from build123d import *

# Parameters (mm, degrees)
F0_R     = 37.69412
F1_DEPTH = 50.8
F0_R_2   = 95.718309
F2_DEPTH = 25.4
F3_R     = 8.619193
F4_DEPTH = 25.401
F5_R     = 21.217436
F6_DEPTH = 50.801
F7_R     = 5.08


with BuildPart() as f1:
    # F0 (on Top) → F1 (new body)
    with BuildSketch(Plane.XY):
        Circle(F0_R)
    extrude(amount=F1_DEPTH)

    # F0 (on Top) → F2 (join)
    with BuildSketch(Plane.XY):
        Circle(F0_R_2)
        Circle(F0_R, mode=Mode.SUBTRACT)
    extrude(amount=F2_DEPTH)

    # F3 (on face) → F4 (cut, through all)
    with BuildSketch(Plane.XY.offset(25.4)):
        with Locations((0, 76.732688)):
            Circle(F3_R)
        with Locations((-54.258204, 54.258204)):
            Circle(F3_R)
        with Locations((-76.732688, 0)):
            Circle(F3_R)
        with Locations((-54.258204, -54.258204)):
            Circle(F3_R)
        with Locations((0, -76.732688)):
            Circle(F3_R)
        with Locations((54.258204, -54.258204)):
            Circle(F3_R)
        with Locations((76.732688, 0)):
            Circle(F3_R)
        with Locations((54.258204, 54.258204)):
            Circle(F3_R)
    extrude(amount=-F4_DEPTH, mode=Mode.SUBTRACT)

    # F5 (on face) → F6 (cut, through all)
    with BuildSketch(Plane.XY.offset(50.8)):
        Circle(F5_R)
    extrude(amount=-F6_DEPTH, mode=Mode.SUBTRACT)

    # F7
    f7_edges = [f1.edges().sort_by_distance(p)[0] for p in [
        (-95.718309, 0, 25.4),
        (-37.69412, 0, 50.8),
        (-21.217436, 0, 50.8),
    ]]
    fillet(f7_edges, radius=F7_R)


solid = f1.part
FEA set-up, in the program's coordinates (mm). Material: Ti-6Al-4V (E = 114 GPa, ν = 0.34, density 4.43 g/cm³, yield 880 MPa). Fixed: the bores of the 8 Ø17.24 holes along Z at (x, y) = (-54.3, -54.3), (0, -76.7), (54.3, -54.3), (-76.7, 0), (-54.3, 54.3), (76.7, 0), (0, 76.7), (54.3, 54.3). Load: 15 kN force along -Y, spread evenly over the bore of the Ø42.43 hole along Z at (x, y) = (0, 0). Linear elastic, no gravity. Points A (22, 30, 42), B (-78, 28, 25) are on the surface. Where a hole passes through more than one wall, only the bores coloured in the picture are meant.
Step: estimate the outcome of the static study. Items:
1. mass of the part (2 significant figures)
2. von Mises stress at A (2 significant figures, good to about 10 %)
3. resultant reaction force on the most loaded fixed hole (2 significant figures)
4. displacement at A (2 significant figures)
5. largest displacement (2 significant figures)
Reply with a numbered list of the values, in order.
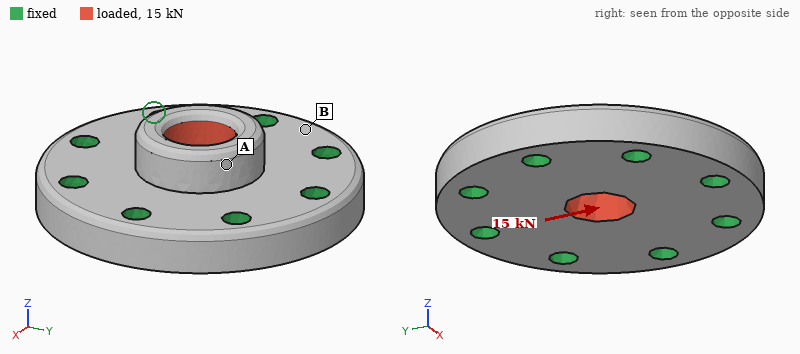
1. 3.2 kg
2. 1.5 MPa
3. 3.2 kN
4. 2.6 µm
5. 3.3 µm
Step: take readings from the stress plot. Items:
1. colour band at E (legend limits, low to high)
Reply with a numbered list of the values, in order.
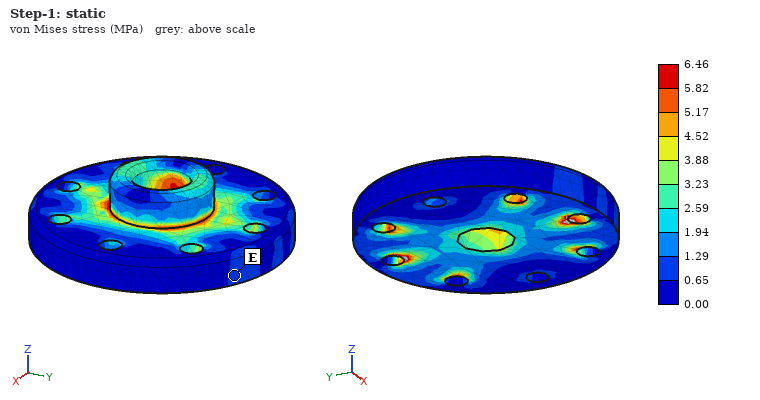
1. 0.65 to 1.29 MPa
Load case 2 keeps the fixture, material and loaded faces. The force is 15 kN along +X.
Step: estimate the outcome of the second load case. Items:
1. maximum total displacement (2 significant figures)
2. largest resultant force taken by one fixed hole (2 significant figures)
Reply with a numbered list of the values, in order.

1. 3.3 µm
2. 3.2 kN
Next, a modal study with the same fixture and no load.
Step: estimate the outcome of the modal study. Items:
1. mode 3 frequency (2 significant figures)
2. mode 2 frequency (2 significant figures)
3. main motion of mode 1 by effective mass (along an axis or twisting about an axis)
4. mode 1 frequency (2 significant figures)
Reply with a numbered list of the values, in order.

1. 12 kHz
2. 12 kHz
3. along Z
4. 8900 Hz
